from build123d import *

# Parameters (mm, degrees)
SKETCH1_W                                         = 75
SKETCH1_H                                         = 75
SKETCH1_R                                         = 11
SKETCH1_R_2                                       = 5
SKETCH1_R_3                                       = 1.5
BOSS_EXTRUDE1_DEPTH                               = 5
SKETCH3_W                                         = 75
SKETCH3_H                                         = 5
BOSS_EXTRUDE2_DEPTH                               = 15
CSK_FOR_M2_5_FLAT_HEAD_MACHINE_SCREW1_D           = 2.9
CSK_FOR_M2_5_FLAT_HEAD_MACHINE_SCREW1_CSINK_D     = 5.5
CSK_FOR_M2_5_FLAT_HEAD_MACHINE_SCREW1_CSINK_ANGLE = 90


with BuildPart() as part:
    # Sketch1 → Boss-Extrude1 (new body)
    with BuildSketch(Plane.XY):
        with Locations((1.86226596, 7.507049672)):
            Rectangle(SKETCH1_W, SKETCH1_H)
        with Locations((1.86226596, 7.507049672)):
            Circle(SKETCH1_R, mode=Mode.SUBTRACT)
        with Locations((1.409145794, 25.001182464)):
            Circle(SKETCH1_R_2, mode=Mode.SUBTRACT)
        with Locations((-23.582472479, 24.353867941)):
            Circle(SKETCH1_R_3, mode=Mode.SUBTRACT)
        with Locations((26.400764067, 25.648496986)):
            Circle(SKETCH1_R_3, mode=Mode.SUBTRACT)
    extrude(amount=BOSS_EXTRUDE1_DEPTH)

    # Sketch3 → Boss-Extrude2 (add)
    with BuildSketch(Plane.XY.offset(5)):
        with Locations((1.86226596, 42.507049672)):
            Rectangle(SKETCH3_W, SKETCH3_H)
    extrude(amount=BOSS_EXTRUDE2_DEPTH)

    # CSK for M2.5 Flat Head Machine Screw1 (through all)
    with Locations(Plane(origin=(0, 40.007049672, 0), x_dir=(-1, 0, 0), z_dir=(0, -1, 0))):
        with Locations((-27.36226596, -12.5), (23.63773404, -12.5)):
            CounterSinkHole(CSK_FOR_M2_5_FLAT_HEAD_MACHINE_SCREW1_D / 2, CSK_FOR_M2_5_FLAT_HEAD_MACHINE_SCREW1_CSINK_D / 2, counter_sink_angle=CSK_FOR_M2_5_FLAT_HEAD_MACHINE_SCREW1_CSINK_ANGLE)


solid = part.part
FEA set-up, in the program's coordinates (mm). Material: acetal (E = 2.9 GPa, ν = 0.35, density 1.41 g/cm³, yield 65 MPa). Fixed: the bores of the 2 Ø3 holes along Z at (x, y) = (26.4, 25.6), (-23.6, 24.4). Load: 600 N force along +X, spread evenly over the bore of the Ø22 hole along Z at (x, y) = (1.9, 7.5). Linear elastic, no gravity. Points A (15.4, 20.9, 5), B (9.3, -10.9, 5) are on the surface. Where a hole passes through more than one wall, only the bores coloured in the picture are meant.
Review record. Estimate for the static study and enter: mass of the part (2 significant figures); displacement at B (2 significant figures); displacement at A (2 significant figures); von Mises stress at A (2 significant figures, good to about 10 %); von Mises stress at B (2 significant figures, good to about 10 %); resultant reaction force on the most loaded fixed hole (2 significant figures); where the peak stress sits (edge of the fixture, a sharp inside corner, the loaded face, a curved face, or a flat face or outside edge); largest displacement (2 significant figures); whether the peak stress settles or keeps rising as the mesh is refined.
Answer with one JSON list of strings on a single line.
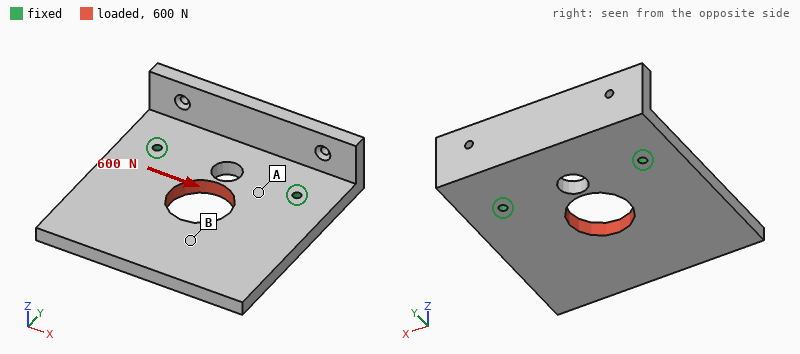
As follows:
["44 g", "0.092 mm", "0.022 mm", "3.5 MPa", "1.5 MPa", "360 N", "edge of the fixture", "0.11 mm", "keeps rising"]
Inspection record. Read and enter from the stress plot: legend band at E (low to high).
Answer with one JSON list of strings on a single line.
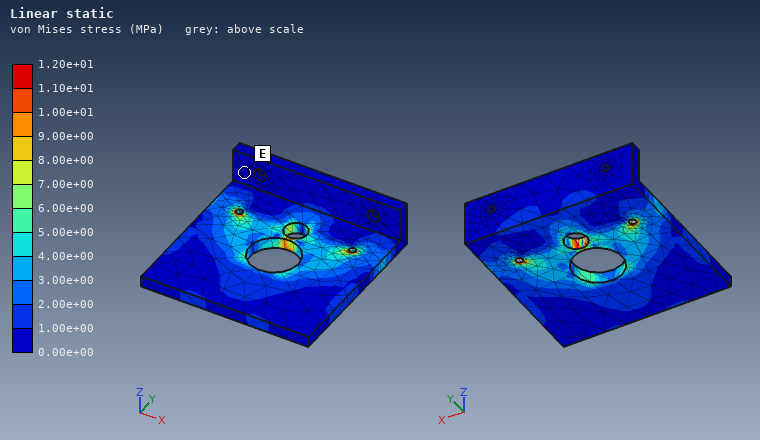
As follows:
["0.00e+00 to 1.00e+00 MPa"]
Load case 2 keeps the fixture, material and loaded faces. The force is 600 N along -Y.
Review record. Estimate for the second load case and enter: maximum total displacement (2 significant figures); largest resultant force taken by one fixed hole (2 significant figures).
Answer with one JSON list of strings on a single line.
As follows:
["53 µm", "310 N"]
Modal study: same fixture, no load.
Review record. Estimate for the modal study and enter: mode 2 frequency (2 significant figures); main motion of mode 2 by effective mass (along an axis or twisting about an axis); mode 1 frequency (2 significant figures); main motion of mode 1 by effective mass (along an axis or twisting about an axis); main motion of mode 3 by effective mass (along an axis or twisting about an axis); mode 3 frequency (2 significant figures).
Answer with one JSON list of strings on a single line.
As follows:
["660 Hz", "twisting about Y", "310 Hz", "along Z", "along Z", "1000 Hz"]
